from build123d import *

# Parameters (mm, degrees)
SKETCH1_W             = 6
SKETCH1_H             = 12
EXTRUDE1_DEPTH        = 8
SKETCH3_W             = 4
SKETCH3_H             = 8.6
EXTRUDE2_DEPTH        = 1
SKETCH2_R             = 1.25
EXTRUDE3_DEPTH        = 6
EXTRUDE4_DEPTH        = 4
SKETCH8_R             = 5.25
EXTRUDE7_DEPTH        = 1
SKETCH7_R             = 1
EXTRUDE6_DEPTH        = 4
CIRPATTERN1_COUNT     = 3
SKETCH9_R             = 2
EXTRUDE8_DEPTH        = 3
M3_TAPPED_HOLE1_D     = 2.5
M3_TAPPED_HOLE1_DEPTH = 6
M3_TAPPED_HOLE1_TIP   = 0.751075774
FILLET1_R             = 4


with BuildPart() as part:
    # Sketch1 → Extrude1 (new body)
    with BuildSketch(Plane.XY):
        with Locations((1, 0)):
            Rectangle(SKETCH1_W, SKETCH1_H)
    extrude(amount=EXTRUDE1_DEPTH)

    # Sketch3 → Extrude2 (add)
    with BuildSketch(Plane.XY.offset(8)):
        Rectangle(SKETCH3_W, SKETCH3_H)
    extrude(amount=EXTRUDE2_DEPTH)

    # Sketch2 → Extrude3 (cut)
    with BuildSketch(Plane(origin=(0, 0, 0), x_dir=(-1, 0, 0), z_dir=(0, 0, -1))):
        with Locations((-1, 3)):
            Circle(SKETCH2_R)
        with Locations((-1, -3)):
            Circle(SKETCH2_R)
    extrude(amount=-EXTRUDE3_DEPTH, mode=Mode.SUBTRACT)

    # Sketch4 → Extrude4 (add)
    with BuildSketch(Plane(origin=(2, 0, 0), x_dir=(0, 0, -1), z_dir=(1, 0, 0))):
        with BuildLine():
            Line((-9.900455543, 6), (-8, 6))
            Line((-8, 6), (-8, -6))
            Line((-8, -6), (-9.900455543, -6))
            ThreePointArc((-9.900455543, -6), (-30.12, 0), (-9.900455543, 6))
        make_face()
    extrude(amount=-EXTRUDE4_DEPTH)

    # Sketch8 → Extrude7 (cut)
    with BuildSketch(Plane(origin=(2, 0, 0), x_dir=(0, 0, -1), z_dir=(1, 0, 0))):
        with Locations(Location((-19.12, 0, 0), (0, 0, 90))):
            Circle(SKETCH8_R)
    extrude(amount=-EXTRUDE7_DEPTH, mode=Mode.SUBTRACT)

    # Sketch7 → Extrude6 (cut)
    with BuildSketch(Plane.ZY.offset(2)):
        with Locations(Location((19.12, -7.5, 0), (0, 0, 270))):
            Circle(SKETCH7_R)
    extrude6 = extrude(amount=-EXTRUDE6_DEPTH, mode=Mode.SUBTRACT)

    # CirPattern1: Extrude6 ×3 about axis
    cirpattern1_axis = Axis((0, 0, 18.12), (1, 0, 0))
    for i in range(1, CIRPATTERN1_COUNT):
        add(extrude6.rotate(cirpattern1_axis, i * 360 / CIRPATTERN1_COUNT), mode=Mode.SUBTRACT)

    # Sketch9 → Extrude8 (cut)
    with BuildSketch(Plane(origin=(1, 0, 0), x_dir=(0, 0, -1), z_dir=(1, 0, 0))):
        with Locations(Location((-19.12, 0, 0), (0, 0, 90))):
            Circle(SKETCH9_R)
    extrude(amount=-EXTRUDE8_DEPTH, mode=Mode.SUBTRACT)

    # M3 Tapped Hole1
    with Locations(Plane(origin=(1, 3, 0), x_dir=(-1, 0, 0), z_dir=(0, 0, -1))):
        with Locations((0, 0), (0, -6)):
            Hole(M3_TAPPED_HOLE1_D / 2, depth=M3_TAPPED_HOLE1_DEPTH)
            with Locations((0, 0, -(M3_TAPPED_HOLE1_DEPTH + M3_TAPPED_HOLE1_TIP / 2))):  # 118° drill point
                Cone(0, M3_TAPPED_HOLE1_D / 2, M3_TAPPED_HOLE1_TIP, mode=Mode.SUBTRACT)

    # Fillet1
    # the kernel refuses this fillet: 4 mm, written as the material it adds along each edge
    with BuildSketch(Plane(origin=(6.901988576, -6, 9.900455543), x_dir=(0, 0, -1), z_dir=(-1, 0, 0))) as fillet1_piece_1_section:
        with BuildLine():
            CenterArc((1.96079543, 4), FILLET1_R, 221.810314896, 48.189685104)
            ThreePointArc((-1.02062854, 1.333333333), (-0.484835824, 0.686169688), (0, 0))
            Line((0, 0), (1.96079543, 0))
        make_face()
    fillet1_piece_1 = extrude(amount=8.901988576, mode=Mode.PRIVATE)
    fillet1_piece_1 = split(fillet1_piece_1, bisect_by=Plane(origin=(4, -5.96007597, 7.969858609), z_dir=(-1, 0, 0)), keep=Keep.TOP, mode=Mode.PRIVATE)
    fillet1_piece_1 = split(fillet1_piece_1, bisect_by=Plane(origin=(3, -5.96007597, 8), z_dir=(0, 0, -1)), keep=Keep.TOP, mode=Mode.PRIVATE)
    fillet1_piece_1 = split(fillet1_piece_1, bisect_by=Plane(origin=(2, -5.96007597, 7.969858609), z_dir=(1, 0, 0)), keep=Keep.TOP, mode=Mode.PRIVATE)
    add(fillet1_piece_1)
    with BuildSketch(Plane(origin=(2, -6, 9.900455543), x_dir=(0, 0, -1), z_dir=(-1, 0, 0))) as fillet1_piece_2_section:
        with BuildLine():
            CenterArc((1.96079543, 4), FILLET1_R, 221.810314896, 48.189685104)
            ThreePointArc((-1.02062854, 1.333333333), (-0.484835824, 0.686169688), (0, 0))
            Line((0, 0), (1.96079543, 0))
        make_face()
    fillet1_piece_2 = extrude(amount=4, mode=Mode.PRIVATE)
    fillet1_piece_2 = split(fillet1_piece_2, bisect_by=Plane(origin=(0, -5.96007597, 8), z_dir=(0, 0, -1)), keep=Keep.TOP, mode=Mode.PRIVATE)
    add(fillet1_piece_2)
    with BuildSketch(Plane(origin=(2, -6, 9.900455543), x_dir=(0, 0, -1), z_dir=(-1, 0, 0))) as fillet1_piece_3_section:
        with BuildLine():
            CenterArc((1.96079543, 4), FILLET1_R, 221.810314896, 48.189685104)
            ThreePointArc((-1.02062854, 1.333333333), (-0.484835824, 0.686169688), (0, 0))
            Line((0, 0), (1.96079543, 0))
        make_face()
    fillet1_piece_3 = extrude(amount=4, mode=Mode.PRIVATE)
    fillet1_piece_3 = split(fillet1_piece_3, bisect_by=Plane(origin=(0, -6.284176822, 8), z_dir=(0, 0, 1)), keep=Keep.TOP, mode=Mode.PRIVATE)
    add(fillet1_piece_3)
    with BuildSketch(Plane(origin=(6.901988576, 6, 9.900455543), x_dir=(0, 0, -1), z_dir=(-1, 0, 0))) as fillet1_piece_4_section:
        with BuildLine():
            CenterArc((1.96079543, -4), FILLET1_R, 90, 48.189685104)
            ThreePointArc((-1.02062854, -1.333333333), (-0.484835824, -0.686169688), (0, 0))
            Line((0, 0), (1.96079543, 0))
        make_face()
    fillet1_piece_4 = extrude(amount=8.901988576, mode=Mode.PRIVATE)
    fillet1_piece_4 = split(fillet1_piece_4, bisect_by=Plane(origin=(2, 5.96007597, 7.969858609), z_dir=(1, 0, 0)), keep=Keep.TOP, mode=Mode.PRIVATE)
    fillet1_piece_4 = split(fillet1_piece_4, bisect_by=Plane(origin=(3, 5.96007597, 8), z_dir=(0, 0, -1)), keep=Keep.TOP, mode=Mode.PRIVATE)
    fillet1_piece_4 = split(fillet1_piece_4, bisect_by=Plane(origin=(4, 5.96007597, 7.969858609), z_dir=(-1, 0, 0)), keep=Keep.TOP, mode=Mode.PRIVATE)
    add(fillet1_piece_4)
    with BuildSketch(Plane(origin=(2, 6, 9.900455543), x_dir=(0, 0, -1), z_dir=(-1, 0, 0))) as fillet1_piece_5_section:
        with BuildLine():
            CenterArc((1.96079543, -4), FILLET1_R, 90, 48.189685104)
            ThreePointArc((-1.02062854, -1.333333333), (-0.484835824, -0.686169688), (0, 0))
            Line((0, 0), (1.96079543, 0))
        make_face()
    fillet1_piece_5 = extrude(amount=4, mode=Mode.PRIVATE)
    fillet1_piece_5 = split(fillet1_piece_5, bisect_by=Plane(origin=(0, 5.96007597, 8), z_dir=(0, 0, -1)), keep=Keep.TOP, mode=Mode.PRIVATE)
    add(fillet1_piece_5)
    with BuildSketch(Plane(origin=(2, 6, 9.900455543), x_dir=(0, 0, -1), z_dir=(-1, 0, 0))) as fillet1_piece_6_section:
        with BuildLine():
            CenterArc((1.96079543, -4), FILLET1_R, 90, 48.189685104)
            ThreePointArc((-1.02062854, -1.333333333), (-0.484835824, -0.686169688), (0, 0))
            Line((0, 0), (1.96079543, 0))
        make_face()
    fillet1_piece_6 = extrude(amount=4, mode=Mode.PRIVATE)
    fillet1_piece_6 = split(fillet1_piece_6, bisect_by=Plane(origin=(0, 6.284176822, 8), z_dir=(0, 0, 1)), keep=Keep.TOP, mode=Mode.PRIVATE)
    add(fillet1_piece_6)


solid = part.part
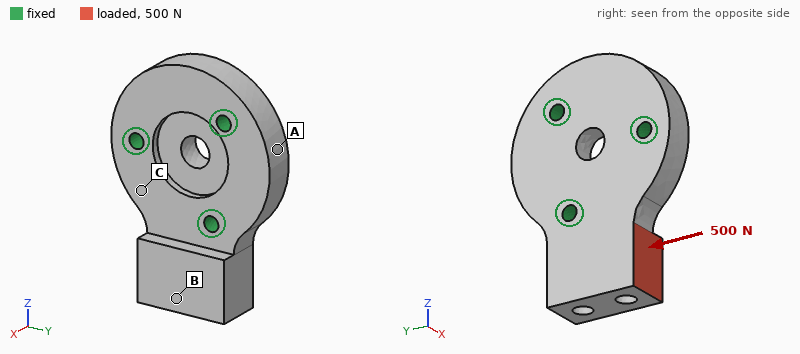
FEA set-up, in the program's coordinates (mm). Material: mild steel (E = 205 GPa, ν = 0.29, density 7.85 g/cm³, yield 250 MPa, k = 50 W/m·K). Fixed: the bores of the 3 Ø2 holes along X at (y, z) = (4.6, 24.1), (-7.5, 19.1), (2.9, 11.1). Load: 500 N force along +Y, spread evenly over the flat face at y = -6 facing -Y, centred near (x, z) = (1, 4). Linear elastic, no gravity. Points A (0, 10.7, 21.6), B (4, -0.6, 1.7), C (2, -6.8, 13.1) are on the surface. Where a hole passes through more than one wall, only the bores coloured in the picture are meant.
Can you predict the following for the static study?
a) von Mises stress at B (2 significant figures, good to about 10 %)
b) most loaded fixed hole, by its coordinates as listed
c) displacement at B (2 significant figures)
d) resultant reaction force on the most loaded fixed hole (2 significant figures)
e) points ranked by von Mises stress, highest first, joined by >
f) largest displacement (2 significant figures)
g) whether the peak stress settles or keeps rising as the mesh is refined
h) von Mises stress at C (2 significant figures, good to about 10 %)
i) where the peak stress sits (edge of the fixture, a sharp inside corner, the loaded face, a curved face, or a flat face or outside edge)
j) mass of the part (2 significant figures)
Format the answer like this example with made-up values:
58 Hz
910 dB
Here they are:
11 MPa
(2.9, 11.1)
2.7 µm
540 N
C > B > A
3.5 µm
keeps rising
17 MPa
edge of the fixture
15 g
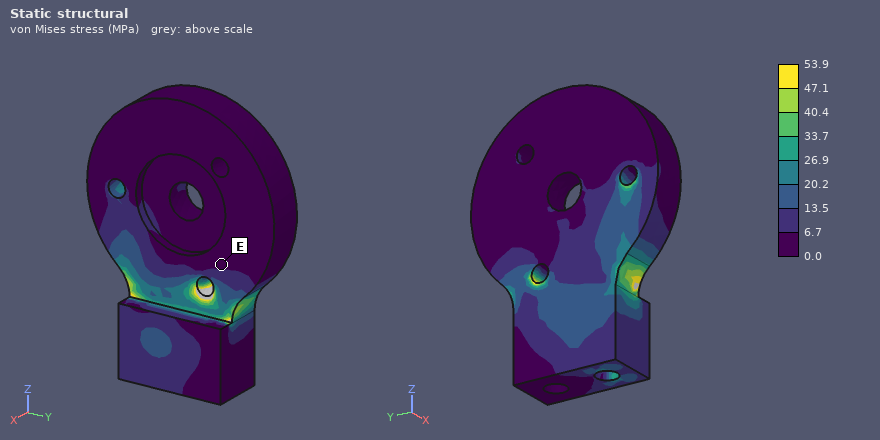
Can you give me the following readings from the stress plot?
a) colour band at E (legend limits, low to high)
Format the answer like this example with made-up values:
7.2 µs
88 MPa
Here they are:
0.0 to 6.7 MPa
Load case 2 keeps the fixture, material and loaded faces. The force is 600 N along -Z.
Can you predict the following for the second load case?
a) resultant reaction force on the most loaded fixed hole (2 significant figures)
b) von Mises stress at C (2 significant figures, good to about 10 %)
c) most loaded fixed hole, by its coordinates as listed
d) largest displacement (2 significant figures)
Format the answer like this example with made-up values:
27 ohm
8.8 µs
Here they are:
460 N
33 MPa
(-7.5, 19.1)
6.0 µm
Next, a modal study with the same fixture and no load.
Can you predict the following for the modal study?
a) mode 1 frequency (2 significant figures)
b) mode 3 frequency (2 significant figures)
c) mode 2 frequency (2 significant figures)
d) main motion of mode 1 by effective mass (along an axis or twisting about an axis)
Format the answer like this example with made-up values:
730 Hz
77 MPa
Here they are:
18 kHz
39 kHz
35 kHz
along X
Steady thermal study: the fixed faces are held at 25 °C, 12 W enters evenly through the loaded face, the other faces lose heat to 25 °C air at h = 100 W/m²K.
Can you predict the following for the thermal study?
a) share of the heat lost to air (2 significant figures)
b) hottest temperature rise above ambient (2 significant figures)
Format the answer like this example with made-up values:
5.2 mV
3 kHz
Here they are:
14 %
59 K
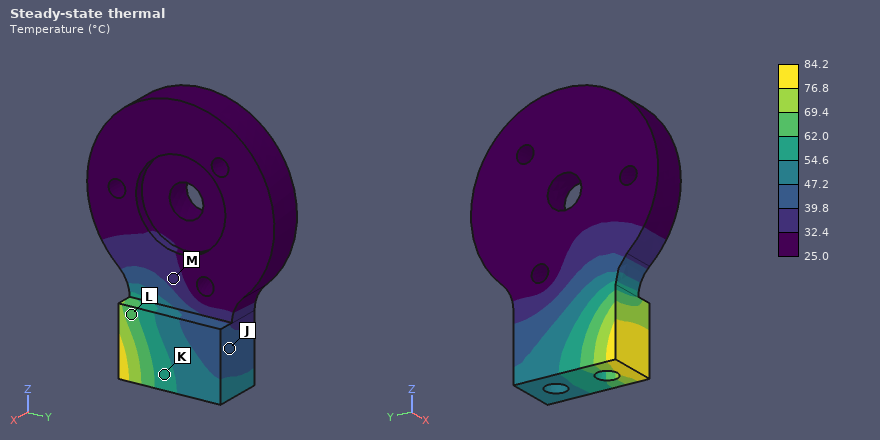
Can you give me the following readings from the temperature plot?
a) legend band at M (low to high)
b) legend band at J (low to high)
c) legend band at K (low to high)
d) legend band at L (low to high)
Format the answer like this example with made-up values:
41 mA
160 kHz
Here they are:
32.4 to 39.8 °C
39.8 to 47.2 °C
54.6 to 62.0 °C
62.0 to 69.4 °C
